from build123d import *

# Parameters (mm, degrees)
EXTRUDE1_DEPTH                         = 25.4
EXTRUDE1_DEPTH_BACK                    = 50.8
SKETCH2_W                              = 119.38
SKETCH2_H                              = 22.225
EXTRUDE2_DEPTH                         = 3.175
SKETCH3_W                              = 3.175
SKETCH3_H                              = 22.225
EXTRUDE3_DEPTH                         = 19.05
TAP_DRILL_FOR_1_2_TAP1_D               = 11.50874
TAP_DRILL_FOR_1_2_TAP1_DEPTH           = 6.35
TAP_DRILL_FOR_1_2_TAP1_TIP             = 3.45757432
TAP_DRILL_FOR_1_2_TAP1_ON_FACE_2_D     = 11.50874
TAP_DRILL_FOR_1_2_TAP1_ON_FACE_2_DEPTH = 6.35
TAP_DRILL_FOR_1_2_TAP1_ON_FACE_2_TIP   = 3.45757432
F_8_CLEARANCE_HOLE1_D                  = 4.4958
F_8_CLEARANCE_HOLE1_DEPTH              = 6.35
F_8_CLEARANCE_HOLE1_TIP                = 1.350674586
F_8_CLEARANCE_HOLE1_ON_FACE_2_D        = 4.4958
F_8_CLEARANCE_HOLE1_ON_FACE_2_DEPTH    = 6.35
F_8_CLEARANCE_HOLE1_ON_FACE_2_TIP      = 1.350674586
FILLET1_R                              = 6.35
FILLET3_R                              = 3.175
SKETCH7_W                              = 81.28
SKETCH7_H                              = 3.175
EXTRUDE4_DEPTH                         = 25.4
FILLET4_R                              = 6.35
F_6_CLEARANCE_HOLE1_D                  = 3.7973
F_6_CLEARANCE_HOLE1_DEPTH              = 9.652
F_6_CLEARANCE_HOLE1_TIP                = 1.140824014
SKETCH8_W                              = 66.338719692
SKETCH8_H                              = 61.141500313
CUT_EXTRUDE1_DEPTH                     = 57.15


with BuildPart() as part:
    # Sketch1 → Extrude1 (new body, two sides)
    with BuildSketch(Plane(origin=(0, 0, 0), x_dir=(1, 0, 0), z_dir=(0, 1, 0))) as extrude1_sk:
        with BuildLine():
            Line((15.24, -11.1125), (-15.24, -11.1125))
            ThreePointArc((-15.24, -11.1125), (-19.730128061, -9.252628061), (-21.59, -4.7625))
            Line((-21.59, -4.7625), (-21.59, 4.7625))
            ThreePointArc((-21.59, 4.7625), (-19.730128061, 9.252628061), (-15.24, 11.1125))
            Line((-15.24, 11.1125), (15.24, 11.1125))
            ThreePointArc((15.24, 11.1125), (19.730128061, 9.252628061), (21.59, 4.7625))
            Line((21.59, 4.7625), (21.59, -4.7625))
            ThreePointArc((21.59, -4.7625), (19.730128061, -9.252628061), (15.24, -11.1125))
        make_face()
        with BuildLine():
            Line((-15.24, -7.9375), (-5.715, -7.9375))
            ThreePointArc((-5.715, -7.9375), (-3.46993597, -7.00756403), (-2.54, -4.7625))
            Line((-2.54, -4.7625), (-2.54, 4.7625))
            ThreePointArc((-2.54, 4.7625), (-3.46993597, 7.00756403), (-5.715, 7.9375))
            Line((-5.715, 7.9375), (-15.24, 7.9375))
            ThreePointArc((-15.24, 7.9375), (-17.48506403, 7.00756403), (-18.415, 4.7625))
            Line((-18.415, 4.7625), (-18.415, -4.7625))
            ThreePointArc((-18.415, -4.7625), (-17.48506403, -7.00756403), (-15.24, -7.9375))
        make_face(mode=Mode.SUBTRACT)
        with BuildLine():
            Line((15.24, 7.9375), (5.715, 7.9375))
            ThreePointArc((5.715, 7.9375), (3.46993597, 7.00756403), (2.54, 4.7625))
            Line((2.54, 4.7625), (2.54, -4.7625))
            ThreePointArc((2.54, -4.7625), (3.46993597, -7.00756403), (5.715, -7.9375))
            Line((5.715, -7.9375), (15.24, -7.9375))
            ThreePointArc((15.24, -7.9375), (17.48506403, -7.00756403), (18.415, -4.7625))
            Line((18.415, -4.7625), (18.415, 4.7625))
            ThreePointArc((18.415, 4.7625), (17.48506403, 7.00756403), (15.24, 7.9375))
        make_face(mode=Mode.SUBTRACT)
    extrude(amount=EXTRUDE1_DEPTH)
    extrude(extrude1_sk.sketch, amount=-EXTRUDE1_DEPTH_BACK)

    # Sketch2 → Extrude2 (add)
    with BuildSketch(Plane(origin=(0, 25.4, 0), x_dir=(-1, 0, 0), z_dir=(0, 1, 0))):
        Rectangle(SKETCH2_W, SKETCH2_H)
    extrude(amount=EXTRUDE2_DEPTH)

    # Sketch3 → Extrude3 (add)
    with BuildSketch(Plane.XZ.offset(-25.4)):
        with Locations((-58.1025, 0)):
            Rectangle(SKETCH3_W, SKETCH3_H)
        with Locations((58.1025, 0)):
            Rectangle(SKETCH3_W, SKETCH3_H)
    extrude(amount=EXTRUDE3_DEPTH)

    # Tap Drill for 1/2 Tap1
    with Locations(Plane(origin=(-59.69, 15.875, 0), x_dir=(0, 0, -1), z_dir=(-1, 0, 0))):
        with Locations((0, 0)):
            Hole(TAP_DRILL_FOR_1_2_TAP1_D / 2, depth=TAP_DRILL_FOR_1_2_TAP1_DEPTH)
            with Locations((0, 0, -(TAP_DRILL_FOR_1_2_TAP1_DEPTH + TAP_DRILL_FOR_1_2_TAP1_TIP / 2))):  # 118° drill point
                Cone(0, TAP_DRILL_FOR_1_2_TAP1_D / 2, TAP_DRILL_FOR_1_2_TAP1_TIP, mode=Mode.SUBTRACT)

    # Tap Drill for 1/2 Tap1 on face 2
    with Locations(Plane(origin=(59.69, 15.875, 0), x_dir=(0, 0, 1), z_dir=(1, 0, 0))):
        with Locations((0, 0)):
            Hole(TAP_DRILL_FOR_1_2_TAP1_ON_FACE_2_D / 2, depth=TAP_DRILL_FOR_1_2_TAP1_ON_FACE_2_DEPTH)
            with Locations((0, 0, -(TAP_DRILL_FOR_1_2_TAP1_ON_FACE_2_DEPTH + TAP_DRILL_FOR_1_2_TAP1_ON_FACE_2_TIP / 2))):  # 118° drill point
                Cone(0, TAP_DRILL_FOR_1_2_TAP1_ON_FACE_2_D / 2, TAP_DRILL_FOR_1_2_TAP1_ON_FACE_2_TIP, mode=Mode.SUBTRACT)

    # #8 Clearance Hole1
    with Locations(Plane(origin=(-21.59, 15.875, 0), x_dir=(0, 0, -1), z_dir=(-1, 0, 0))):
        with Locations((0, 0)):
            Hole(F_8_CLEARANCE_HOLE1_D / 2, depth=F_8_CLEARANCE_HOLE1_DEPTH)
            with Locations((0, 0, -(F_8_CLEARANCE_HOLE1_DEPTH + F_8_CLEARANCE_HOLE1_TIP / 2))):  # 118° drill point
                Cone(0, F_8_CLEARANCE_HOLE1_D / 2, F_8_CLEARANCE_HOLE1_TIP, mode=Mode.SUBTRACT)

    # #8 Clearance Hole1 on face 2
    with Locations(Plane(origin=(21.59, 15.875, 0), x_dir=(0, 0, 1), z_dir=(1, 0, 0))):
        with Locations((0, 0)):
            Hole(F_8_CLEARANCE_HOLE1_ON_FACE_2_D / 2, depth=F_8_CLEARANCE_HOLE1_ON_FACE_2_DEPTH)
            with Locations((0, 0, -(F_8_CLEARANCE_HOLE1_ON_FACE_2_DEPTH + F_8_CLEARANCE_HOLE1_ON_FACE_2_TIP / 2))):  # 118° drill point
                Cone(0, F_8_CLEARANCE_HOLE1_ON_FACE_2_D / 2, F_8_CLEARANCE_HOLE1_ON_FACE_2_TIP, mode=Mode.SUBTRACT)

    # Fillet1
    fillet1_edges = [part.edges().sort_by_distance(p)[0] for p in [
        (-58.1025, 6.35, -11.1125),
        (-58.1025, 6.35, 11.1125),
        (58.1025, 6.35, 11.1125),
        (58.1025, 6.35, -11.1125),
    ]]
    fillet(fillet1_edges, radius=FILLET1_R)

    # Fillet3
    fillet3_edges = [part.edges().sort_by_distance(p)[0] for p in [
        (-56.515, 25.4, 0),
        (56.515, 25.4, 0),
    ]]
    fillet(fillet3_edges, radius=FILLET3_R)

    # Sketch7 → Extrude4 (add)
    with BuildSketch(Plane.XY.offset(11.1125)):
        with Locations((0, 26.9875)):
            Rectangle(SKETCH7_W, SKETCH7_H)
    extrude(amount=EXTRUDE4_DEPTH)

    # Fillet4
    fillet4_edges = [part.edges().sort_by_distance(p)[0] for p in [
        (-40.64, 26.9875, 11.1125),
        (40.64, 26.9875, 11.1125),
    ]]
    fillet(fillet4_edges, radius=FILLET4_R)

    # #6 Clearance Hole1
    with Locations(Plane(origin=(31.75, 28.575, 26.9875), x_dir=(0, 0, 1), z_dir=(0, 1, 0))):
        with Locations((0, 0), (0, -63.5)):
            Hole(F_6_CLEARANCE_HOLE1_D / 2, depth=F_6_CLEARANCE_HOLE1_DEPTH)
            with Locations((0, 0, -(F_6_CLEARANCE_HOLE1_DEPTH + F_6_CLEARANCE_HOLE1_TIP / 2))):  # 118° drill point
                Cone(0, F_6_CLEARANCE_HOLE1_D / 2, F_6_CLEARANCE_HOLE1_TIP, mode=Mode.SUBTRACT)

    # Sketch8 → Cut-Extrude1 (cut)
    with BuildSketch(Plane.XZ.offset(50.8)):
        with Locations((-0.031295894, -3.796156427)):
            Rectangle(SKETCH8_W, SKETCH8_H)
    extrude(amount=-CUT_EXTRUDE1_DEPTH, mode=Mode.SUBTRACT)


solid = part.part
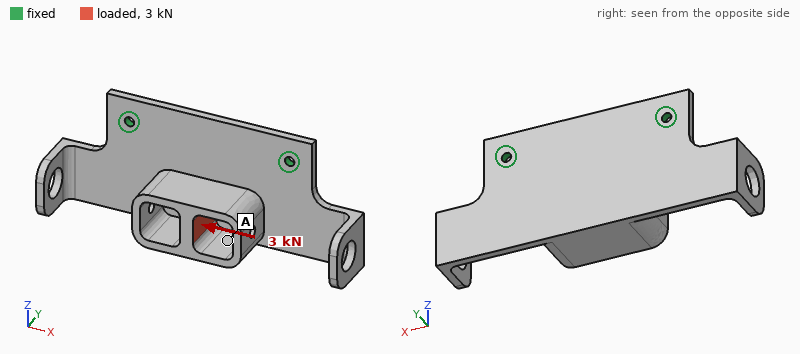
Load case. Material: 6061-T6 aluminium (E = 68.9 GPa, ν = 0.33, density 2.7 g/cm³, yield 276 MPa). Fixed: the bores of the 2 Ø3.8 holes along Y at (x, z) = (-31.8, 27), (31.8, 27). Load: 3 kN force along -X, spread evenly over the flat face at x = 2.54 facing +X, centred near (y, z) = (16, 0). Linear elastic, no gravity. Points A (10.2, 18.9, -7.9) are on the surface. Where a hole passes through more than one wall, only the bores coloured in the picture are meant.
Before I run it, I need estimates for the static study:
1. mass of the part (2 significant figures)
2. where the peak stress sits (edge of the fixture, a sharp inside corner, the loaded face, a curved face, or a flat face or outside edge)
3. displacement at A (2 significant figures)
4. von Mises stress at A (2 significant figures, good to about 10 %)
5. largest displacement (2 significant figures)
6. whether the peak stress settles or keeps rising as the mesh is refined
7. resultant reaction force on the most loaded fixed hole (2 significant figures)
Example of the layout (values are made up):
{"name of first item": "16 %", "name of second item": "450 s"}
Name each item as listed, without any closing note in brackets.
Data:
{"mass of the part": "68 g", "where the peak stress sits": "edge of the fixture", "displacement at A": "0.11 mm", "von Mises stress at A": "17 MPa", "largest displacement": "0.30 mm", "whether the peak stress settles or keeps rising as the mesh is refined": "keeps rising", "resultant reaction force on the most loaded fixed hole": "2.0 kN"}
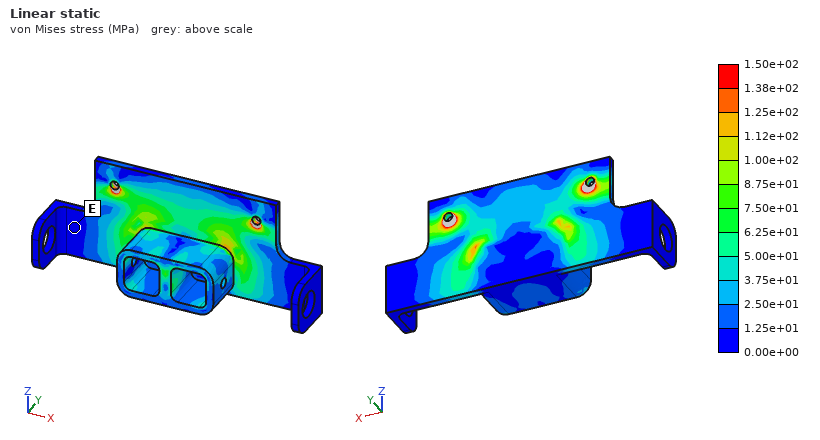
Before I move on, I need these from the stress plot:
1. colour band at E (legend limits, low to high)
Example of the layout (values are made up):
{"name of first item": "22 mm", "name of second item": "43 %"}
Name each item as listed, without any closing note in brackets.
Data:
{"colour band at E": "0.00e+00 to 1.25e+01 MPa"}
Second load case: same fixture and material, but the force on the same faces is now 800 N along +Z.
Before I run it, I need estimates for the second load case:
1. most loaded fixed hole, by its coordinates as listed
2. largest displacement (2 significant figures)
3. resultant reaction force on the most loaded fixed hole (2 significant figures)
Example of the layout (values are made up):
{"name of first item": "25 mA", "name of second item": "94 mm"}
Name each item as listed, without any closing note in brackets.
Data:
{"most loaded fixed hole, by its coordinates as listed": "(31.8, 27)", "largest displacement": "0.53 mm", "resultant reaction force on the most loaded fixed hole": "480 N"}
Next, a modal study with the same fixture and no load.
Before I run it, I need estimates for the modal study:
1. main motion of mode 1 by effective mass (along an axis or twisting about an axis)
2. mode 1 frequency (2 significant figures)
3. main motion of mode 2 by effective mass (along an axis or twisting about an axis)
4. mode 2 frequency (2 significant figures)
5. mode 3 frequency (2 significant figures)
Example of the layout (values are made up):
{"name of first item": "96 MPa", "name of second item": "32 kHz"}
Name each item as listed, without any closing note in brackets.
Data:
{"main motion of mode 1 by effective mass": "along Y", "mode 1 frequency": "770 Hz", "main motion of mode 2 by effective mass": "twisting about Z", "mode 2 frequency": "1200 Hz", "mode 3 frequency": "1400 Hz"}
